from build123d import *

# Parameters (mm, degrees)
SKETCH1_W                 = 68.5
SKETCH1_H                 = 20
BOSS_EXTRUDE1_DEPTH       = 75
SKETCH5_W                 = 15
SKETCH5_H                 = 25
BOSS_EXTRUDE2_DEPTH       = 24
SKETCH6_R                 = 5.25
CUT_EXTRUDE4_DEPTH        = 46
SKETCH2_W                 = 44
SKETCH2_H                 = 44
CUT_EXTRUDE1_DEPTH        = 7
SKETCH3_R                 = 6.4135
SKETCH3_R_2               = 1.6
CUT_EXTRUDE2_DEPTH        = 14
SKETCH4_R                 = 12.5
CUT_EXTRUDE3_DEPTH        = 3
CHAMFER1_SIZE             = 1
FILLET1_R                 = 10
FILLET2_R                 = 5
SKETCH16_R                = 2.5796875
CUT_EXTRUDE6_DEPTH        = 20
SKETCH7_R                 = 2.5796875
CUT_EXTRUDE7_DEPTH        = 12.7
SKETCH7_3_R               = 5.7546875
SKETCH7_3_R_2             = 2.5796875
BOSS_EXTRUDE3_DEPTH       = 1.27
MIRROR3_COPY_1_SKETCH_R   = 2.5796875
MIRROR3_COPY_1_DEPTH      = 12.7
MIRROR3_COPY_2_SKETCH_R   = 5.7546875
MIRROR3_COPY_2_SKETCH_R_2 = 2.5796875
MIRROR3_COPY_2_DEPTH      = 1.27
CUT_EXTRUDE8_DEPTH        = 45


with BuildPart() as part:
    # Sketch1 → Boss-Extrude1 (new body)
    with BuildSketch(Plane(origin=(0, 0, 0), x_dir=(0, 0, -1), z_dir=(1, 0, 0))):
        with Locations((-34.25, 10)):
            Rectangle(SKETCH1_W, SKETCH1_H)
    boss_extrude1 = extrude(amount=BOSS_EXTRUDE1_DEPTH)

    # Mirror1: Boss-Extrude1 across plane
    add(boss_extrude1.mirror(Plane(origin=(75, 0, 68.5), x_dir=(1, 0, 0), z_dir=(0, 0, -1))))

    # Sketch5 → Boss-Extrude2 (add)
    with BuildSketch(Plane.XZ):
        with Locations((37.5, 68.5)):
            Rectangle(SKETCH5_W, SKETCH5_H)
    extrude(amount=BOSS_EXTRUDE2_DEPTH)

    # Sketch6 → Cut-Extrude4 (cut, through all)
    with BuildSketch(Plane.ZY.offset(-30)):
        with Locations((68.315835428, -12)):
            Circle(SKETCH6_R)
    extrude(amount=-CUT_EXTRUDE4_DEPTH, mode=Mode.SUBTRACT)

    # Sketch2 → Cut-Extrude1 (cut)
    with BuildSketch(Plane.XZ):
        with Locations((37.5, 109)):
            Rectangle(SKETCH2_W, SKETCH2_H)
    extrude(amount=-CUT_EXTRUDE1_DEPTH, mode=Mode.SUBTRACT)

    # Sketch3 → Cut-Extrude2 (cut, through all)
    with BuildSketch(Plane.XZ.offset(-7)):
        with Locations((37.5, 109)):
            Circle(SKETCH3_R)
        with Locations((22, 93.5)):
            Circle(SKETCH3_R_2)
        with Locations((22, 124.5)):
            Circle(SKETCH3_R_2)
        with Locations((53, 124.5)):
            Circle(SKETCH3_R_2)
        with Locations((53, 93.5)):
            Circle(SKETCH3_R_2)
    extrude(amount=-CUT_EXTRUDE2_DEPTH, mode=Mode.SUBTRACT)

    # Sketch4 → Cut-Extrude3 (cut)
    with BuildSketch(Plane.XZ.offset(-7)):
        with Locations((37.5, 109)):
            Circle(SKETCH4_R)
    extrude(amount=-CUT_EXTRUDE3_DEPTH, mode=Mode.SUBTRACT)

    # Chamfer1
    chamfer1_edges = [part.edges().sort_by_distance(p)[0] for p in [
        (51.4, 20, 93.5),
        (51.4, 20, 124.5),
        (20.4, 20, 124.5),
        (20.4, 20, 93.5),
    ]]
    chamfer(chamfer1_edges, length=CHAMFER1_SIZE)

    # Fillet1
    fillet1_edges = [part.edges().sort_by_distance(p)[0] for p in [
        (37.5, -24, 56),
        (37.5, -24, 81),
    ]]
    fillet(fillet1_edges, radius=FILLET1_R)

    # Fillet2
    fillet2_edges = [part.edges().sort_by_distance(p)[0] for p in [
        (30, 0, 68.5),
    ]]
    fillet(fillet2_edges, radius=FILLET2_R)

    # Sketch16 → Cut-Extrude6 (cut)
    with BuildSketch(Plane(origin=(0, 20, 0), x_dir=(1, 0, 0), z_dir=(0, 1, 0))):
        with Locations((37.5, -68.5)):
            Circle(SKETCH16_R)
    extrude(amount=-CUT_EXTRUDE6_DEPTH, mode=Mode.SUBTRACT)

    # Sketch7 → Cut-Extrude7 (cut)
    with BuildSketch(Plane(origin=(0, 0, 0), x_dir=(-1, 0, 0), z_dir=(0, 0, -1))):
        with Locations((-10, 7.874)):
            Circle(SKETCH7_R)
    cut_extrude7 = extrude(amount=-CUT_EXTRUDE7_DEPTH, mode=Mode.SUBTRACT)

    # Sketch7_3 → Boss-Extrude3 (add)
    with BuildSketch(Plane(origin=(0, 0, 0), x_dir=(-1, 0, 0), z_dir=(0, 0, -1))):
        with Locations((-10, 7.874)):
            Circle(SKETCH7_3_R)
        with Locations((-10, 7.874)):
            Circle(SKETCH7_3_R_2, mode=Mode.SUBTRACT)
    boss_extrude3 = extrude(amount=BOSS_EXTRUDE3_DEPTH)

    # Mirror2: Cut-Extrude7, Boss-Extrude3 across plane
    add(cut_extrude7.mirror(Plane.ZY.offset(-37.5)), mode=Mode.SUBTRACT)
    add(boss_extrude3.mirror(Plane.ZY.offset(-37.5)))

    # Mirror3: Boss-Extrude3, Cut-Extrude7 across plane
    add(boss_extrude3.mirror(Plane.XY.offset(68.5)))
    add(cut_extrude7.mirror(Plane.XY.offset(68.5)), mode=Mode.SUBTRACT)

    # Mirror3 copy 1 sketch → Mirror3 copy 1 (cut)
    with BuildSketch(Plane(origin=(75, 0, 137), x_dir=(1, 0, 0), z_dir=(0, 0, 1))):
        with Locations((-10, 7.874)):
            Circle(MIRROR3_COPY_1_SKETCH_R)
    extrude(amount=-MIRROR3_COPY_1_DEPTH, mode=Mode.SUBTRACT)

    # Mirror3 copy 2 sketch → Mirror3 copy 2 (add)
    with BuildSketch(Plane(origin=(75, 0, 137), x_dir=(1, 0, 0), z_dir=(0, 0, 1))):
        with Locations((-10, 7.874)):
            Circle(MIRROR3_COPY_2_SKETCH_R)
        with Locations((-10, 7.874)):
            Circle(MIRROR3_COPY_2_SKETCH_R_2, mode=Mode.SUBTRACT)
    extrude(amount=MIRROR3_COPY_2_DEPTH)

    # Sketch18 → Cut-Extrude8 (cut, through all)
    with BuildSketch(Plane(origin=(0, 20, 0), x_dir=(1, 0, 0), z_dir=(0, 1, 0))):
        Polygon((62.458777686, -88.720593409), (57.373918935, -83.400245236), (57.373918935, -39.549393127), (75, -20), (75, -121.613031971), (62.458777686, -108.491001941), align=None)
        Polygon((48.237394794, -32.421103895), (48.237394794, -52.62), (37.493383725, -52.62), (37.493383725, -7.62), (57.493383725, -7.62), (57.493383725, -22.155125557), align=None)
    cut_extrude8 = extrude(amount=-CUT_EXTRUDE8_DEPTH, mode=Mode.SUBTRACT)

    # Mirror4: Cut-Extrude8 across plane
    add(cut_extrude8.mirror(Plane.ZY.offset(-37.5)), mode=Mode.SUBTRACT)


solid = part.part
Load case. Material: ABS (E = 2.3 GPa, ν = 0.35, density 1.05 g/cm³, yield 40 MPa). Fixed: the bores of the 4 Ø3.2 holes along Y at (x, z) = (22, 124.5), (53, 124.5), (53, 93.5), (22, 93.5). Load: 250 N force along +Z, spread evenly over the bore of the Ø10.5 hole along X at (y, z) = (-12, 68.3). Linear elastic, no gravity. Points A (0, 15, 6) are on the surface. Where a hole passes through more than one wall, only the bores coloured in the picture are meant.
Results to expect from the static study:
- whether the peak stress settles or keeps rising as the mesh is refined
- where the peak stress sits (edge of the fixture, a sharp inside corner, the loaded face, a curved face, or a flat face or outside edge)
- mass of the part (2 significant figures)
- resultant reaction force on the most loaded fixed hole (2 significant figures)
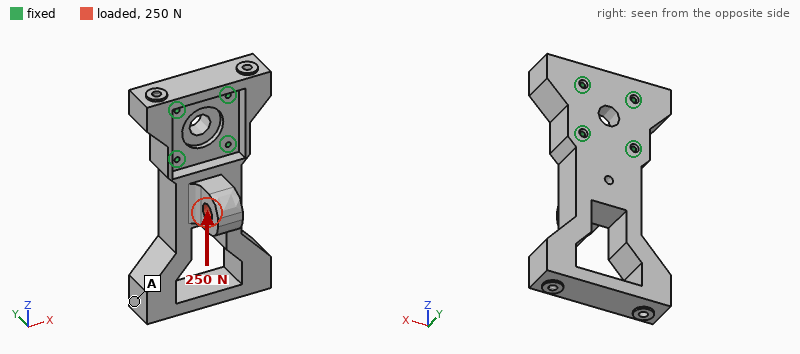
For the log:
keeps rising
edge of the fixture
120 g
130 N
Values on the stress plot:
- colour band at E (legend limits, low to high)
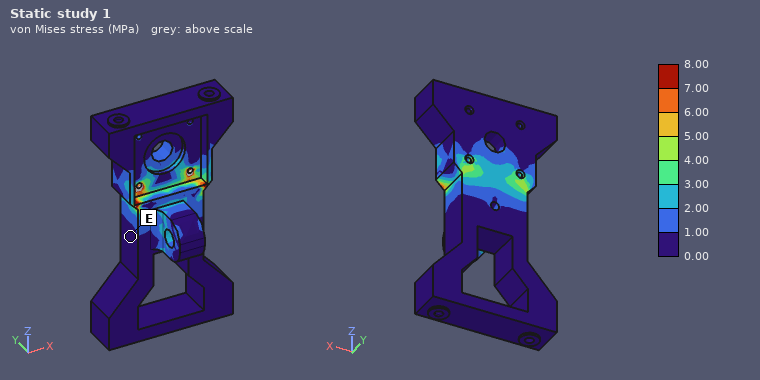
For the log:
0.00 to 1.00 MPa
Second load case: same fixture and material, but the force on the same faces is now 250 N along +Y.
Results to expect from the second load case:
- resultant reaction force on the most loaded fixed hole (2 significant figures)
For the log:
170 N
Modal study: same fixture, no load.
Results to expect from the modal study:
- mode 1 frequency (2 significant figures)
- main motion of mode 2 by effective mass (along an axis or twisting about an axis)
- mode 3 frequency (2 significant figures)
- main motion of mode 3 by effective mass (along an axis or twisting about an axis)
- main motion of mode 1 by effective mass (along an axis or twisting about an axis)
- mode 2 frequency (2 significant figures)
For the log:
330 Hz
along X
720 Hz
twisting about Z
along Y
440 Hz
